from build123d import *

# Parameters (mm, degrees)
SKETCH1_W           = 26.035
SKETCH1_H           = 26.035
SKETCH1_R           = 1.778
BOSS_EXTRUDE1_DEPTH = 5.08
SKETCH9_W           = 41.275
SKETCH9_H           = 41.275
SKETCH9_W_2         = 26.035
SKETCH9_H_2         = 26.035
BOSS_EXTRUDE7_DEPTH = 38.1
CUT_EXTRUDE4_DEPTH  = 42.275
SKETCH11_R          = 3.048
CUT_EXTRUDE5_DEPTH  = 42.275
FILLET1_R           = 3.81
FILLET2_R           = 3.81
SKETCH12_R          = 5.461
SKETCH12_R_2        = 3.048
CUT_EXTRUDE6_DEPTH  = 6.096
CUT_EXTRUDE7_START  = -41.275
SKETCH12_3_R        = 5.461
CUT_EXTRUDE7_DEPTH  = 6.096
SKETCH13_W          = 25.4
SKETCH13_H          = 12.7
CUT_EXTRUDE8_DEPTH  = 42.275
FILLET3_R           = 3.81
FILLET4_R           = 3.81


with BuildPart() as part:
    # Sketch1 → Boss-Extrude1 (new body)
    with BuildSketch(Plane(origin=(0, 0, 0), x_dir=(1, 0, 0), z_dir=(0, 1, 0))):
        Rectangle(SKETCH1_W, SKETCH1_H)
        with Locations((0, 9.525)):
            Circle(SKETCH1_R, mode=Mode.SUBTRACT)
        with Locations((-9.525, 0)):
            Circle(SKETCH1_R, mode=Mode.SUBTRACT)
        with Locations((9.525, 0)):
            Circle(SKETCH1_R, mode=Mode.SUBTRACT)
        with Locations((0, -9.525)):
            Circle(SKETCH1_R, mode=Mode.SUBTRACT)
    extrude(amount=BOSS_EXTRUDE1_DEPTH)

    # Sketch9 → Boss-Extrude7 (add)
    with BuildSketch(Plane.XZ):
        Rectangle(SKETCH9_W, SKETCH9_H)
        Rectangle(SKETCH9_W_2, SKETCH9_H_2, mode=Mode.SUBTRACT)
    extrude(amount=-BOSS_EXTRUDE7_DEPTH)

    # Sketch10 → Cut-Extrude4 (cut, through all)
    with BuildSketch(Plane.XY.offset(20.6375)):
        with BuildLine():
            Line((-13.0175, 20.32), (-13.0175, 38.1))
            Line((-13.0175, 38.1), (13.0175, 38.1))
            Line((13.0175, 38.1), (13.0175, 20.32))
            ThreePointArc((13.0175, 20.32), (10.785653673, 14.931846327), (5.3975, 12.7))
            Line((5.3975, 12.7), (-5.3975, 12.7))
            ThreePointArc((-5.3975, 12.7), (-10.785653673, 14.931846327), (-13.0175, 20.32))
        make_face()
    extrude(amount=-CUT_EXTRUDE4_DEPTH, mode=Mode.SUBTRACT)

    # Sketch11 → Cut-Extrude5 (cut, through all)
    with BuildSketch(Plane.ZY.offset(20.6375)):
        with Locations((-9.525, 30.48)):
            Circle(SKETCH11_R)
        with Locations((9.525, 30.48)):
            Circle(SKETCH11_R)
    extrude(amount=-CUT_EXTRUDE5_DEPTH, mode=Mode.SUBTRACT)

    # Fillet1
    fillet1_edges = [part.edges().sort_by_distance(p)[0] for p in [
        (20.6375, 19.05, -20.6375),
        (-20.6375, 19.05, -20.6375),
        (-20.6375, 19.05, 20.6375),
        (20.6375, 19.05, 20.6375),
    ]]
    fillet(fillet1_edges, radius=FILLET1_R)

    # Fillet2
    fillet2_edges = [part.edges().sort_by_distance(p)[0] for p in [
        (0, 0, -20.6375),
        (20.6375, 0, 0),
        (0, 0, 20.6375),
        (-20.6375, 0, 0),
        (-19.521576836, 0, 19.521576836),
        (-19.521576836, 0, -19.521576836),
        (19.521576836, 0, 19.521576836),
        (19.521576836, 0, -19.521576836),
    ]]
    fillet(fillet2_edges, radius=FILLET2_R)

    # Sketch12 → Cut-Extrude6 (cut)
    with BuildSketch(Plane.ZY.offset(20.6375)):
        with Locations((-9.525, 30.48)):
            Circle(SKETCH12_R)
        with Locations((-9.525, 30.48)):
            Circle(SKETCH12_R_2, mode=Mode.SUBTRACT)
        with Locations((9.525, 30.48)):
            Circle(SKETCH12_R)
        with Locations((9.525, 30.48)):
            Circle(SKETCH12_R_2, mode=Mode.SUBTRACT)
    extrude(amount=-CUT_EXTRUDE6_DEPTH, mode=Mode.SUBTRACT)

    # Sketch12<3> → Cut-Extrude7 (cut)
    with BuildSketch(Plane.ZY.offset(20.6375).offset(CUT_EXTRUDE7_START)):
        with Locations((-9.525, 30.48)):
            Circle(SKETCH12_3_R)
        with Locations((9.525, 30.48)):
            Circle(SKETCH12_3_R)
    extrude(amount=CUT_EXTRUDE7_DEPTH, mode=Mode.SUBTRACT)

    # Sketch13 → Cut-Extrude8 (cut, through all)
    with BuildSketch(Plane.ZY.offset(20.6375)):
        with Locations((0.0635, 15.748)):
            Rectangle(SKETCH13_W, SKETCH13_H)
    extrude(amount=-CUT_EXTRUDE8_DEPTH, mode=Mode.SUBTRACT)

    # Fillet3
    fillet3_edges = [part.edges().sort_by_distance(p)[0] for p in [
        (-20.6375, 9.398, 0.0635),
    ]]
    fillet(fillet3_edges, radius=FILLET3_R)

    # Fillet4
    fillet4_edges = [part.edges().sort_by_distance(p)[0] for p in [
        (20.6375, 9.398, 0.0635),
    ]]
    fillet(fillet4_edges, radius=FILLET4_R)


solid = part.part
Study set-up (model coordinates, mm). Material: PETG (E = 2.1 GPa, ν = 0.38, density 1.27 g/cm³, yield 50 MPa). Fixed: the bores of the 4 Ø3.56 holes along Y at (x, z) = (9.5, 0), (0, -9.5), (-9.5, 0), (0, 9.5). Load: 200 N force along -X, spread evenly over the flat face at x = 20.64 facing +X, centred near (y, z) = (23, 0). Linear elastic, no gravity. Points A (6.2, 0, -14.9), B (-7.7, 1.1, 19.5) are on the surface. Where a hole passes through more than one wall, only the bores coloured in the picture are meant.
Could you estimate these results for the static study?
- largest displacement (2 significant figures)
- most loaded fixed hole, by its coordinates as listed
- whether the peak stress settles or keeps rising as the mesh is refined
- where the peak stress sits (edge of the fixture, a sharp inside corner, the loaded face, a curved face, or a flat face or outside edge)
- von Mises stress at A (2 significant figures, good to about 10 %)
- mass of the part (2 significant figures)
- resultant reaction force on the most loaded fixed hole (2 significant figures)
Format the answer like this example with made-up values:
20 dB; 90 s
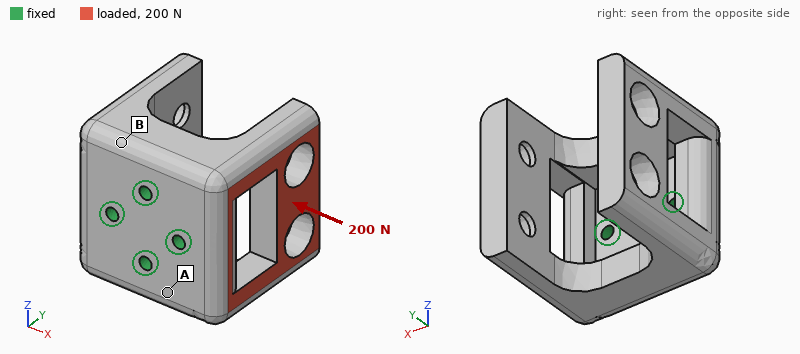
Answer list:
0.77 mm; (9.5, 0); keeps rising; edge of the fixture; 3.6 MPa; 31 g; 170 N
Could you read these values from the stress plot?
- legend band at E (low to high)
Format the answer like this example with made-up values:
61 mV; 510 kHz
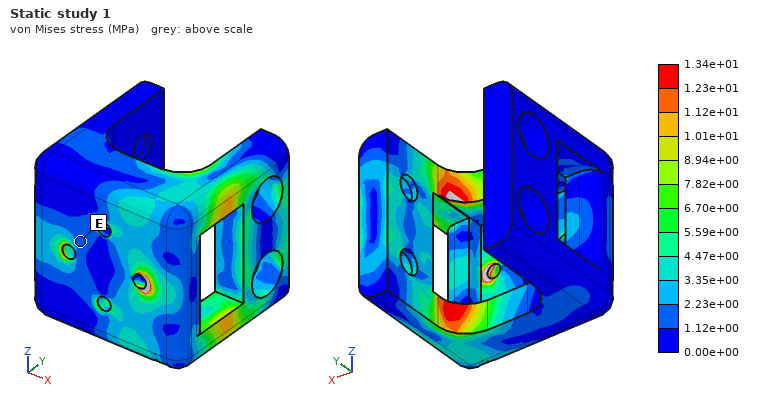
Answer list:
1.12e+00 to 2.23e+00 MPa
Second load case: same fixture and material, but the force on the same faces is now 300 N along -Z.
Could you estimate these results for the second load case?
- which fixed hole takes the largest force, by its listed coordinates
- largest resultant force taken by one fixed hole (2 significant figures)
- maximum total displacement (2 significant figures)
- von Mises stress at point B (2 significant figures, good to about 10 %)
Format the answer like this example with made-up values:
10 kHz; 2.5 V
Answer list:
(9.5, 0); 310 N; 0.69 mm; 3.4 MPa
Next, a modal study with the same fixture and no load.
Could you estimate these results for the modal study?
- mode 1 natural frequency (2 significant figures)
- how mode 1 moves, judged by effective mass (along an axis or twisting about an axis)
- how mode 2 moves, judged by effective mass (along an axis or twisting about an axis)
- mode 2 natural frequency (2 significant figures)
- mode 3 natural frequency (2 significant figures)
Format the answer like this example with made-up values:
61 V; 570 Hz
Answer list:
1000 Hz; along X; along Z; 1200 Hz; 1200 Hz
